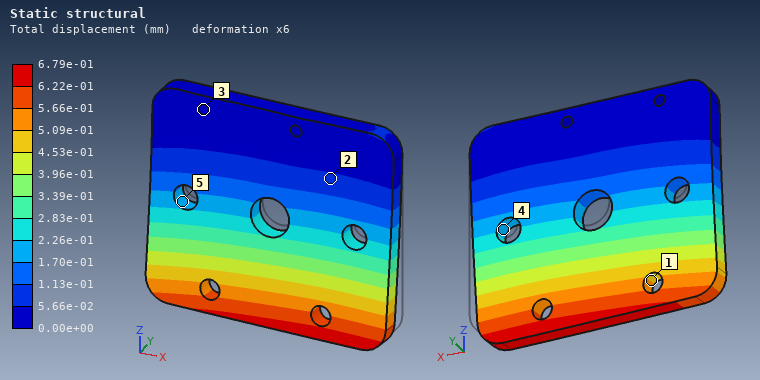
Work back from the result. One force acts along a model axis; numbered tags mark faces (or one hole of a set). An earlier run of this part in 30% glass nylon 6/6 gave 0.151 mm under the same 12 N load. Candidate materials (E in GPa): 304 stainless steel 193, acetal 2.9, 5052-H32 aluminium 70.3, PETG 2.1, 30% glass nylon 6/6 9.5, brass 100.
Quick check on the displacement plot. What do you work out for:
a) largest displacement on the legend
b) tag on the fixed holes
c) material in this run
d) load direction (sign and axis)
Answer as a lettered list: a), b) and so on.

a) 6.79e-01 mm
b) 3
c) PETG
d) -Y
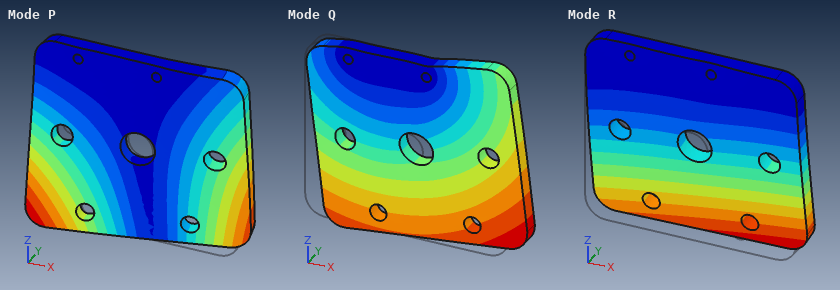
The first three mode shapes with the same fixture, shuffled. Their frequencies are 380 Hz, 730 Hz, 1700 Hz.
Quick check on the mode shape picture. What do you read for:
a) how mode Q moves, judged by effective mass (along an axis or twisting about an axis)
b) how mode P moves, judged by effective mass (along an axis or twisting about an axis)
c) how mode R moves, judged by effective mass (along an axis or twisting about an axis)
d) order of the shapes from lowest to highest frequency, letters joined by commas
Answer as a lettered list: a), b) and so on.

a) along X
b) twisting about Z
c) along Y
d) R, P, Q
